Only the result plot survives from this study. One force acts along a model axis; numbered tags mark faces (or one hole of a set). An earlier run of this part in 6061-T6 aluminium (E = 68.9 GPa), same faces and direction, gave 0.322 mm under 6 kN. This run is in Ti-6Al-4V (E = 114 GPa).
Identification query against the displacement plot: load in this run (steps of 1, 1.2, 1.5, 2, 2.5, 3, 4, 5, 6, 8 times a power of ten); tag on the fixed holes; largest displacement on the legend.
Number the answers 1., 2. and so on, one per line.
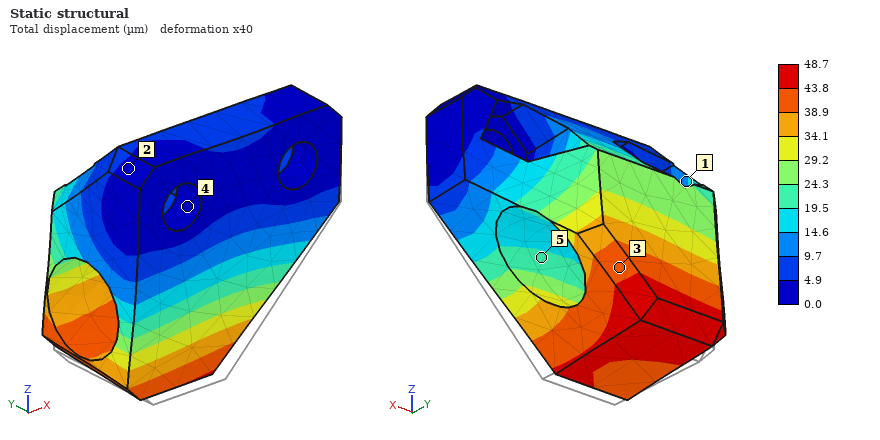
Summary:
1. 1.5 kN
2. 4
3. 48.7 µm
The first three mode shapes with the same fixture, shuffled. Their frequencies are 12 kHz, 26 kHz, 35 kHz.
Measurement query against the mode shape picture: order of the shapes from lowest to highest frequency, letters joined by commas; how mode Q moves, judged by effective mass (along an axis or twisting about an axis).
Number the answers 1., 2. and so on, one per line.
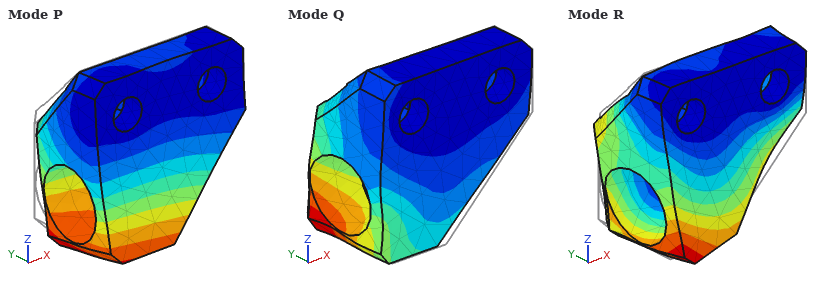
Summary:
1. P, Q, R
2. along X
